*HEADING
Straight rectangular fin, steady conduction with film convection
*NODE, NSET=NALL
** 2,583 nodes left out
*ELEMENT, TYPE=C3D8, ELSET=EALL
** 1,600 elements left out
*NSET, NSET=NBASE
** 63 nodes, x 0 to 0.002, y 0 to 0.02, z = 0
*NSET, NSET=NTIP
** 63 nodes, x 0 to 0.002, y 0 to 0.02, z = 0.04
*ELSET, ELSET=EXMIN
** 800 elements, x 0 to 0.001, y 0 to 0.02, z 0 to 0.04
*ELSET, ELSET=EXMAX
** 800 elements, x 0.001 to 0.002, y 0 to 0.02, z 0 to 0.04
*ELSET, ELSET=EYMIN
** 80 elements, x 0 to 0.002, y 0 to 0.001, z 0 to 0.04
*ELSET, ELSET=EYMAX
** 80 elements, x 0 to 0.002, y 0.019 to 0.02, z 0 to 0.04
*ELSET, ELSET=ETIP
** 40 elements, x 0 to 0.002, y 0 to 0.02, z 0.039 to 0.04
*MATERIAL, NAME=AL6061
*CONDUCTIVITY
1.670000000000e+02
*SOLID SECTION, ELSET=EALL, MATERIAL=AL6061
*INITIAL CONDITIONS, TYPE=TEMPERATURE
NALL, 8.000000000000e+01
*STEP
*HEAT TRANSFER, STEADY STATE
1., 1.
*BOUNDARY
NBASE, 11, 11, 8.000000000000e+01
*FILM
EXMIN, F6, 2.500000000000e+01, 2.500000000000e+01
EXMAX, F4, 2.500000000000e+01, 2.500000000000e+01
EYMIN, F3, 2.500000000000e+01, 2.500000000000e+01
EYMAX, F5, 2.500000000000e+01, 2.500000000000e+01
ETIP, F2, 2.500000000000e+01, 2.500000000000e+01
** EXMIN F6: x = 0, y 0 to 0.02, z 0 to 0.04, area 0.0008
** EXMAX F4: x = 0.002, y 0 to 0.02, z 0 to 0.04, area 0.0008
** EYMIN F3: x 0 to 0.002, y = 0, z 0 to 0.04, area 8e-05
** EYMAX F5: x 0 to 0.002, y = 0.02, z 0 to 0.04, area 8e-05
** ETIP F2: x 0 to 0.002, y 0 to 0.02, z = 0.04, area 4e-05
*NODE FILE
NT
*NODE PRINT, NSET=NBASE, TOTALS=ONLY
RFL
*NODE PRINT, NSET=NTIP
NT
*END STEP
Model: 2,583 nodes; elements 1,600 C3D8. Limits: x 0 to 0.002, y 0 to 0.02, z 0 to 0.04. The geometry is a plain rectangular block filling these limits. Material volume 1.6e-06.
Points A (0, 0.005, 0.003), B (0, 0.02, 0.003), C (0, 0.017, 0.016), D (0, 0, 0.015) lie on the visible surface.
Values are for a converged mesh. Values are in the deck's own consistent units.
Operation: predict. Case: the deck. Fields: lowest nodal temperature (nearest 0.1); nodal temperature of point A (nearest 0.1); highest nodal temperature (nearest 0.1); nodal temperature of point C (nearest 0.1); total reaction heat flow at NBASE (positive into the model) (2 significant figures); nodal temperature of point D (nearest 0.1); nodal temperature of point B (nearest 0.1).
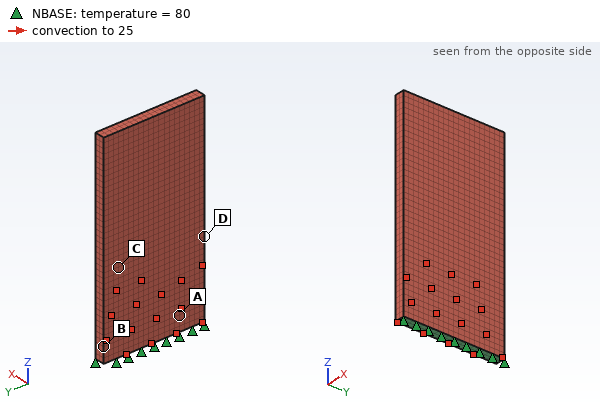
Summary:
73.2
79.0
80.0
75.7
2.3
75.9
79.0
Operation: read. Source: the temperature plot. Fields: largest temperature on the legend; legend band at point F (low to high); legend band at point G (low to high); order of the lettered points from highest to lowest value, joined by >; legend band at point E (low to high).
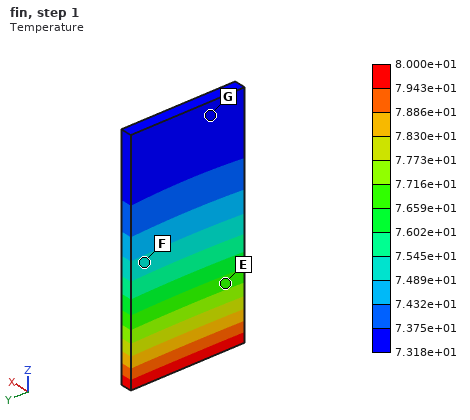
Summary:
8.000e+01
7.489e+01 to 7.545e+01
7.318e+01 to 7.375e+01
E > F > G
7.659e+01 to 7.716e+01
